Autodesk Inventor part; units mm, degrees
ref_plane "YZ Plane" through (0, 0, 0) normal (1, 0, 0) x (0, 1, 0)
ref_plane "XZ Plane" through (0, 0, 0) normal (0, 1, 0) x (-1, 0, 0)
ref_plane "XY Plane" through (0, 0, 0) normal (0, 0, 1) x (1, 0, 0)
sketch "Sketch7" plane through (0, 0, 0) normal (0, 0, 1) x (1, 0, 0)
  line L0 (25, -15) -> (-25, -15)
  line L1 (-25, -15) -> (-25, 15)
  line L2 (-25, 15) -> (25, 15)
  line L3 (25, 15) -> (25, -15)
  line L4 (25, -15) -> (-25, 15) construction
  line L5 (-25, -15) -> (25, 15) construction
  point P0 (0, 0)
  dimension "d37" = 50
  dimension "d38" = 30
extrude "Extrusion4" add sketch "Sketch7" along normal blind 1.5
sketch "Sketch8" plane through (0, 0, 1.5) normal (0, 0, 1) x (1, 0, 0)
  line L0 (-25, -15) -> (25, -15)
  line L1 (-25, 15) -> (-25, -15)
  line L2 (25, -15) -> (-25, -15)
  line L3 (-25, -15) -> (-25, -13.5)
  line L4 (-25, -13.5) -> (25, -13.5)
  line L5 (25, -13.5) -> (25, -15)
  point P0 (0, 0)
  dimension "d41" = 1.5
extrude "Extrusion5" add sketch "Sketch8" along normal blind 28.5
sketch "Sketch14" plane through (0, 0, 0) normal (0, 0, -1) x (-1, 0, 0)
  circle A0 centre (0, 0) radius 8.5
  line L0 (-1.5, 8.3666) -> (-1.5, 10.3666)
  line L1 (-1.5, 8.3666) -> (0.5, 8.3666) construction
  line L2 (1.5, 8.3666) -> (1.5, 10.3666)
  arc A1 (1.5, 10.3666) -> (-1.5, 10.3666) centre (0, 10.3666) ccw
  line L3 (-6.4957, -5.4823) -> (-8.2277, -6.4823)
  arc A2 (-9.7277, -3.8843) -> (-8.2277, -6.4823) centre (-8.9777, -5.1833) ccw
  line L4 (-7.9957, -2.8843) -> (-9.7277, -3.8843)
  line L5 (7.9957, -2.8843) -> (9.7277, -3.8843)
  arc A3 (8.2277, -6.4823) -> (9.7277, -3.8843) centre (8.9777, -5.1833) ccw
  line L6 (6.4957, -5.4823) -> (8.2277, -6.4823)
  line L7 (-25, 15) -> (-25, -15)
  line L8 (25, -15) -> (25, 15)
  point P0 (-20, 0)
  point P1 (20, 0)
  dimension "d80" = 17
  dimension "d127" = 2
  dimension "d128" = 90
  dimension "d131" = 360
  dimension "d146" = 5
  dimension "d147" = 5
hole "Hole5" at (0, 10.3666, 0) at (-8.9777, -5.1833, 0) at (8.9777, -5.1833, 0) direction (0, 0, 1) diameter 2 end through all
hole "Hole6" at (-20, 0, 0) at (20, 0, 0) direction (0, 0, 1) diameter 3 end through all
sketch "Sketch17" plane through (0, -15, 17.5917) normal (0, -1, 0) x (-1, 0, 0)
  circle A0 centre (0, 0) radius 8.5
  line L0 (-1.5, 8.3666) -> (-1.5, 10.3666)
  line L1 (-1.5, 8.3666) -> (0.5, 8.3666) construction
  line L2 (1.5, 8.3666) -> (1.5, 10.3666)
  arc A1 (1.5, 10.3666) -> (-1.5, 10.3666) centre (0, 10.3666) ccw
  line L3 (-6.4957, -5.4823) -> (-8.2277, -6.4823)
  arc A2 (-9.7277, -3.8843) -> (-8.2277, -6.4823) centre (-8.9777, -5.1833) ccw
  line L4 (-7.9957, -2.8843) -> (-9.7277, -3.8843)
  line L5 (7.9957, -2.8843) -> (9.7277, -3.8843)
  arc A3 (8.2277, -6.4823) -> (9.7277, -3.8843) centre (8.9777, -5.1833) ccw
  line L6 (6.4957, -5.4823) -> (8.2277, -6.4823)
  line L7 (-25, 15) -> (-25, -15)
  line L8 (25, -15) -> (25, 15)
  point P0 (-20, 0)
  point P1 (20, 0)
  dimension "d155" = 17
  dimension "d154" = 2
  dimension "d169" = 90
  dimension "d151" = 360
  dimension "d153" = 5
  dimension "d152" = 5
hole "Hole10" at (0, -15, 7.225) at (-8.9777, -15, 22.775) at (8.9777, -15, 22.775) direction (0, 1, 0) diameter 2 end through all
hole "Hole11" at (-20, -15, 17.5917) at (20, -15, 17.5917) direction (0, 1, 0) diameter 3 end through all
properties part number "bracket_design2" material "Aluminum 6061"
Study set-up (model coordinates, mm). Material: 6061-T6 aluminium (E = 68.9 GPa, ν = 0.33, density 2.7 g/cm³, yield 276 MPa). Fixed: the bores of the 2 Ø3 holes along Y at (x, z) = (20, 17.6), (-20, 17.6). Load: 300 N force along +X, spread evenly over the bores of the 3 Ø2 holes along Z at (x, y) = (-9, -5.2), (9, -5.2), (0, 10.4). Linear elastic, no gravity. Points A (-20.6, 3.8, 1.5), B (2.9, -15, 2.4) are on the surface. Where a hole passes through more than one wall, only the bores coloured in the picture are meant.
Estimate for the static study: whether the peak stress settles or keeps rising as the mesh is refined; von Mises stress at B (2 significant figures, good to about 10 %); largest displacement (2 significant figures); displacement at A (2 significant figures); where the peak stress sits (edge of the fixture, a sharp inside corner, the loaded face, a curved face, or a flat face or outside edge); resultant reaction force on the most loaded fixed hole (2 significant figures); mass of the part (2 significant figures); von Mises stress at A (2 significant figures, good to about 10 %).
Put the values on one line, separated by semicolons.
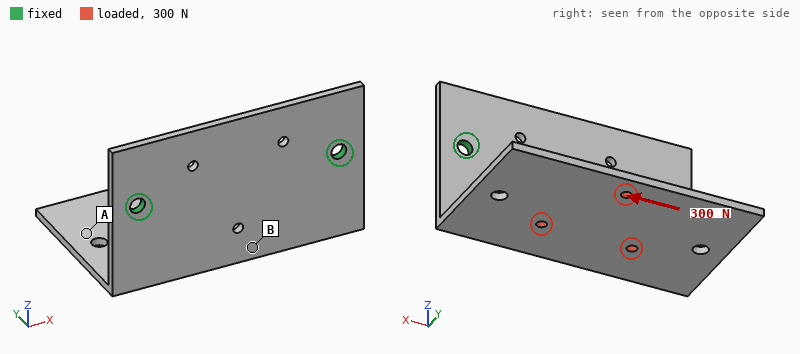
keeps rising; 48 MPa; 0.53 mm; 0.37 mm; edge of the fixture; 220 N; 12 g; 19 MPa
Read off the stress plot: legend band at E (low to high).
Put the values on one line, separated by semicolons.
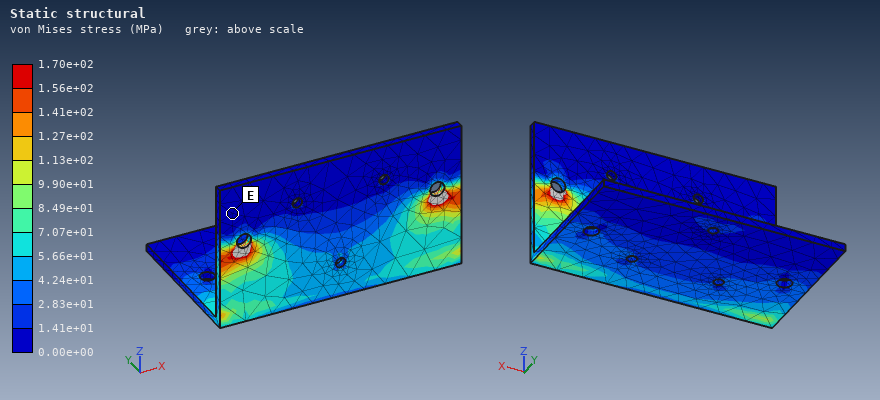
0.00e+00 to 1.41e+01 MPa
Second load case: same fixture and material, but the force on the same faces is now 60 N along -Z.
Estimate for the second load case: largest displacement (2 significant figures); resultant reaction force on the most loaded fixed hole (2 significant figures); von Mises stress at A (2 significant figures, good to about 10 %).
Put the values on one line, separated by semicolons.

0.64 mm; 31 N; 7.3 MPa
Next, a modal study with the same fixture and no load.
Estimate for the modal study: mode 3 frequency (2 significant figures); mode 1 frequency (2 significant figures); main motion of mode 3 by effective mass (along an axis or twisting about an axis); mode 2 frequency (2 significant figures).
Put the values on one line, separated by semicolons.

2100 Hz; 720 Hz; along Y; 1500 Hz
